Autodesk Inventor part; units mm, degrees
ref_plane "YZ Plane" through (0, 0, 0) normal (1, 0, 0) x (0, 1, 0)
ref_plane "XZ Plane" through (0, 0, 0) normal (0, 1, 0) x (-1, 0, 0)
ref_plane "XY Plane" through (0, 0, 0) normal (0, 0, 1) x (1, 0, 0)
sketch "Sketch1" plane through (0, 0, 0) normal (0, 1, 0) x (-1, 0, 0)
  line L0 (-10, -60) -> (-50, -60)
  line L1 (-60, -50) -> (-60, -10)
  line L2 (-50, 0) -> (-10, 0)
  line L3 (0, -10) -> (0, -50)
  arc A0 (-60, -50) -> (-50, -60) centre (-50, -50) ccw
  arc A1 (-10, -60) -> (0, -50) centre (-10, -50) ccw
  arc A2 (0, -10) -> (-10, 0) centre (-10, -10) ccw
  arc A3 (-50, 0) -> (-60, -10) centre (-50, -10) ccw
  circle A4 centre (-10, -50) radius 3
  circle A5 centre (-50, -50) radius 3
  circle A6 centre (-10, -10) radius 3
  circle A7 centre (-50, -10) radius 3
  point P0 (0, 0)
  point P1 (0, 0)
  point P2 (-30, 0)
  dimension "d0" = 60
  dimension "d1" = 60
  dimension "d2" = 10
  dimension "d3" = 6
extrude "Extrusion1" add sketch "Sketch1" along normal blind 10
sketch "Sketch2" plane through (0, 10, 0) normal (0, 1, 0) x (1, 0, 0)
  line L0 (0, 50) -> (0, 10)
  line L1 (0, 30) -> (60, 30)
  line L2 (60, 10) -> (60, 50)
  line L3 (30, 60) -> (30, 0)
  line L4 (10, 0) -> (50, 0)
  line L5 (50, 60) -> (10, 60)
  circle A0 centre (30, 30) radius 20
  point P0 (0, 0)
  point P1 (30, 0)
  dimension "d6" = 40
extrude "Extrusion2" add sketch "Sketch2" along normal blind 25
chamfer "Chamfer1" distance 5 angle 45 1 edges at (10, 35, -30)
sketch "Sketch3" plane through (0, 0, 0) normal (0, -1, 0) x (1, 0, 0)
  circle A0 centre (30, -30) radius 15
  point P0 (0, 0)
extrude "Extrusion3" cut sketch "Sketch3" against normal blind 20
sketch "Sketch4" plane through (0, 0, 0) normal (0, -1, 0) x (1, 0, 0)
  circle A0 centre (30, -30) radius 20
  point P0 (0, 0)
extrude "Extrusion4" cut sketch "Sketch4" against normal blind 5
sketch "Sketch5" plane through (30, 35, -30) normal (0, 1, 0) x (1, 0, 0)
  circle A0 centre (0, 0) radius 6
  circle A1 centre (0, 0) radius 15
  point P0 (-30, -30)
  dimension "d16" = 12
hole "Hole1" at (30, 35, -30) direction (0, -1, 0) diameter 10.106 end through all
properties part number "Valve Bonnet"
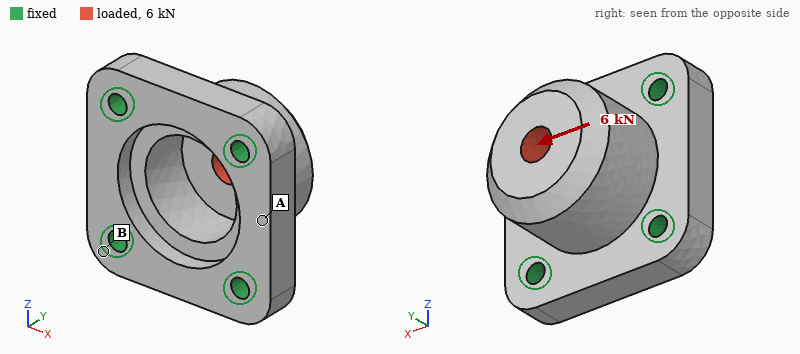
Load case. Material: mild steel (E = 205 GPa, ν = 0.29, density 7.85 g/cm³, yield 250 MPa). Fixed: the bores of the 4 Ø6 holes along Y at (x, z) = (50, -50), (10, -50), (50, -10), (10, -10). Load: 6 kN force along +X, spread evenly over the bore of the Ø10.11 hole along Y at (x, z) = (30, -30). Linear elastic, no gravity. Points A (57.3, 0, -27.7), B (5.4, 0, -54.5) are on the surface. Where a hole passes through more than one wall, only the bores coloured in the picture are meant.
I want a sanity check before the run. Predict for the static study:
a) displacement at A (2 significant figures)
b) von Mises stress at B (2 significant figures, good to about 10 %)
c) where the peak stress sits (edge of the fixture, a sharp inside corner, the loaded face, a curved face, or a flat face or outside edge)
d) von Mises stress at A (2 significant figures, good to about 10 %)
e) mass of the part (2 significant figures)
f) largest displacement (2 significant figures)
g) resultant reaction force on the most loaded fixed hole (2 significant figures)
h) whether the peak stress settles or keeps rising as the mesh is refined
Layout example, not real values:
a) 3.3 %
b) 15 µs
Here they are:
a) 2.5 µm
b) 8.4 MPa
c) edge of the fixture
d) 21 MPa
e) 360 g
f) 9.8 µm
g) 2.4 kN
h) keeps rising
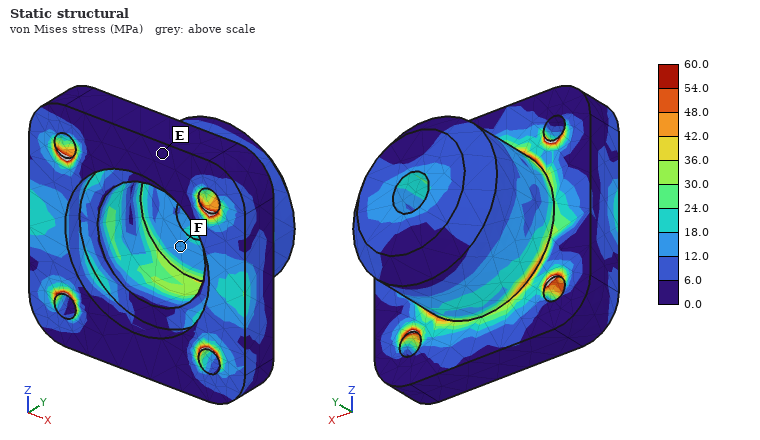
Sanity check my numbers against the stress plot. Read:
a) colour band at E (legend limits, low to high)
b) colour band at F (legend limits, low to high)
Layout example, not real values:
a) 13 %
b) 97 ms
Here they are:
a) 0.0 to 6.0 MPa
b) 12.0 to 18.0 MPa
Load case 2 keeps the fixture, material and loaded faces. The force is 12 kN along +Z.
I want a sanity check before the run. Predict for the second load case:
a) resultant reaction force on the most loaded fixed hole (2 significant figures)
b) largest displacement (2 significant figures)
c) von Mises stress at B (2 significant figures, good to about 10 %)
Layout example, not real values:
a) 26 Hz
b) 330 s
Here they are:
a) 4.7 kN
b) 20 µm
c) 17 MPa
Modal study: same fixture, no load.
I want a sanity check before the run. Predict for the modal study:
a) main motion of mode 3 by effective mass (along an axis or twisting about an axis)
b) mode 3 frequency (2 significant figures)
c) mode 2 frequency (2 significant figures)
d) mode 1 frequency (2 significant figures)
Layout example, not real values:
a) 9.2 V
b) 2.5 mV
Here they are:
a) along Y
b) 17 kHz
c) 12 kHz
d) 12 kHz
